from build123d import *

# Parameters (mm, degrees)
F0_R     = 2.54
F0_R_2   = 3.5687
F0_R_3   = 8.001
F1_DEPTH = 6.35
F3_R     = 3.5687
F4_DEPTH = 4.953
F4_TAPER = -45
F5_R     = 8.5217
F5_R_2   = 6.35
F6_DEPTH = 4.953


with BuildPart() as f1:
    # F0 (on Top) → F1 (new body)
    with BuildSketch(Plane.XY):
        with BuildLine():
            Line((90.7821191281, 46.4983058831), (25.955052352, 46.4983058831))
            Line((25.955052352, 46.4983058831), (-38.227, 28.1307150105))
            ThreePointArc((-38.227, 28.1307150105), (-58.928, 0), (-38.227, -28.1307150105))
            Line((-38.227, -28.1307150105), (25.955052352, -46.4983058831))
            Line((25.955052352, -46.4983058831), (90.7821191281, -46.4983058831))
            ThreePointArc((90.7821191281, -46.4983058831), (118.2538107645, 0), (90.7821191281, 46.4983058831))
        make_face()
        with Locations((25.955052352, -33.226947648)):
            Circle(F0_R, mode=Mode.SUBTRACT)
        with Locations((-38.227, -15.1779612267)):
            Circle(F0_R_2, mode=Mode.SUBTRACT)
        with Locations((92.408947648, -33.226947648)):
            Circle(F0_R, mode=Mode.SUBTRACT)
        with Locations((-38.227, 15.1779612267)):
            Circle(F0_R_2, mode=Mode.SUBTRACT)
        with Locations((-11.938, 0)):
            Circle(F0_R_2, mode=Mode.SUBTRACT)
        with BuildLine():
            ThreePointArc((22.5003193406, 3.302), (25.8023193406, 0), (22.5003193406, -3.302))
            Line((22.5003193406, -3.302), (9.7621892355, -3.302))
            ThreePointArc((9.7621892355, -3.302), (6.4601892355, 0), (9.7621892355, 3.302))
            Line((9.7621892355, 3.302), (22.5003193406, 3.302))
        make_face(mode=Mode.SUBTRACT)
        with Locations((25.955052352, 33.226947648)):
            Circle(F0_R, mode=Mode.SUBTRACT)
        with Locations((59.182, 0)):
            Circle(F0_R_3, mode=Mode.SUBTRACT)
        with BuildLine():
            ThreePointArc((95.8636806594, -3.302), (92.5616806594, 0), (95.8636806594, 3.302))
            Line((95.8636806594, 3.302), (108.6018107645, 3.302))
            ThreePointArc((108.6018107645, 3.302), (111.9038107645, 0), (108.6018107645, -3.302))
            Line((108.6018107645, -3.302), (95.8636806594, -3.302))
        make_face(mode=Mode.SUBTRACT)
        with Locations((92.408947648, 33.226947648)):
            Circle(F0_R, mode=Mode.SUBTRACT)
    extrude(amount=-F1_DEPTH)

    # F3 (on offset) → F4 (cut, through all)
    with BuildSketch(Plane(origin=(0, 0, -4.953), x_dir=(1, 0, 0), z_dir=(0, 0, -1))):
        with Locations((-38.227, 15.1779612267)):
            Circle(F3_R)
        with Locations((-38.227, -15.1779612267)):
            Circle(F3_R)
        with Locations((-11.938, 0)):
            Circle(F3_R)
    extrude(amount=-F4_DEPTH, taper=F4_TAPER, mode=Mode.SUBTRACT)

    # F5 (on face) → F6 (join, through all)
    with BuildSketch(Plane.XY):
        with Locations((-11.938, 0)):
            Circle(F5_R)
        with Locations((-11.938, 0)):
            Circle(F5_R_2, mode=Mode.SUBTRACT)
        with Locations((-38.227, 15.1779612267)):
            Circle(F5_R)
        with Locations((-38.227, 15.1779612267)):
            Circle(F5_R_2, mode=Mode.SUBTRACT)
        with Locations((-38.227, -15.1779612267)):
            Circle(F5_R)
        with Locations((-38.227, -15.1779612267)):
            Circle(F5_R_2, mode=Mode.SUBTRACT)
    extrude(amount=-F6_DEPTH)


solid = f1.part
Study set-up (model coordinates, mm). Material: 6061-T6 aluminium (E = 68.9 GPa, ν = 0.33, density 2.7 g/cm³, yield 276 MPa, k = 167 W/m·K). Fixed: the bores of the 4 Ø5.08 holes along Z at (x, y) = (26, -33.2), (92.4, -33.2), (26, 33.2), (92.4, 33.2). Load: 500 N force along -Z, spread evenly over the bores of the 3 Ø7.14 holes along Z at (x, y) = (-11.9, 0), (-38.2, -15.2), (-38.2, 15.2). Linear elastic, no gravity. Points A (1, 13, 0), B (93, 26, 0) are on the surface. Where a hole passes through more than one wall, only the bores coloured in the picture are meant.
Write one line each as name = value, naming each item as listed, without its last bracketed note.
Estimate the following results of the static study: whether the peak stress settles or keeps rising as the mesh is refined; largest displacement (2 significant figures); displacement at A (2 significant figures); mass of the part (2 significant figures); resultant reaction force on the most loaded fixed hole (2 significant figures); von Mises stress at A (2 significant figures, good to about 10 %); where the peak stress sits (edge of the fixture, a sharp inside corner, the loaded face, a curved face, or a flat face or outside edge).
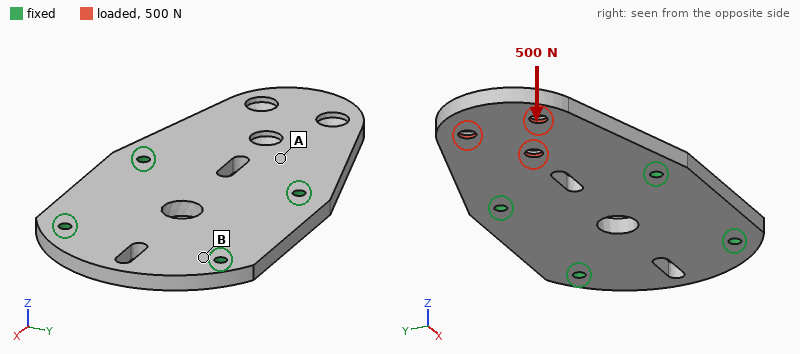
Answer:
whether the peak stress settles or keeps rising as the mesh is refined = keeps rising
largest displacement = 0.56 mm
displacement at A = 0.095 mm
mass of the part = 220 g
resultant reaction force on the most loaded fixed hole = 320 N
von Mises stress at A = 29 MPa
where the peak stress sits = edge of the fixture
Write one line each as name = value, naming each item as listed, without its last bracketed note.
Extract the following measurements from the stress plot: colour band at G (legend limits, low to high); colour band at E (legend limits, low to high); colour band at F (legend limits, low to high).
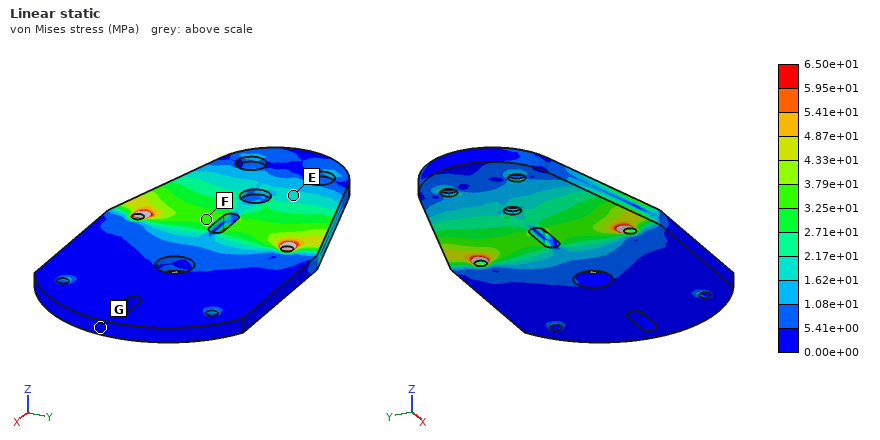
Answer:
colour band at G = 0.00e+00 to 5.41e+00 MPa
colour band at E = 1.62e+01 to 2.17e+01 MPa
colour band at F = 3.25e+01 to 3.79e+01 MPa
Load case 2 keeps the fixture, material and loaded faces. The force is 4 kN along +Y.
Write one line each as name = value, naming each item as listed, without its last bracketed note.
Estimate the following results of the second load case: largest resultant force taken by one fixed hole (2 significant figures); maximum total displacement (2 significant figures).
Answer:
largest resultant force taken by one fixed hole = 3.5 kN
maximum total displacement = 80 µm
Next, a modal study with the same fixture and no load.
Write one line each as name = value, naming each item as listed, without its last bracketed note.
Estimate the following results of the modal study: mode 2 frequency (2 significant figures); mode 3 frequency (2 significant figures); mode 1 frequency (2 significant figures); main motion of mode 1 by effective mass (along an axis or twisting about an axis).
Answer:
mode 2 frequency = 3000 Hz
mode 3 frequency = 4300 Hz
mode 1 frequency = 880 Hz
main motion of mode 1 by effective mass = along Z
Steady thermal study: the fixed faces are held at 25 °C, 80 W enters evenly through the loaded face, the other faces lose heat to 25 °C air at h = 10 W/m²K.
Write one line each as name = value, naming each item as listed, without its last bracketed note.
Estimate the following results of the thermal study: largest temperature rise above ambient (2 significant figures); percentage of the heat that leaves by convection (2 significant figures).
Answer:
largest temperature rise above ambient = 78 K
percentage of the heat that leaves by convection = 7.0 %
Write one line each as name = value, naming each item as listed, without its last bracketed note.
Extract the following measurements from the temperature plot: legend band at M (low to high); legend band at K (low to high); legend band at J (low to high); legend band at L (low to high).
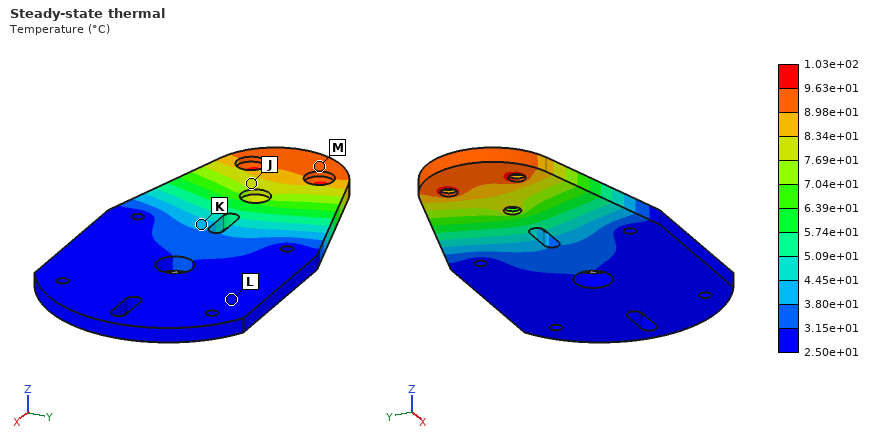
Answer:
legend band at M = 8.98e+01 to 9.63e+01 °C
legend band at K = 3.80e+01 to 4.45e+01 °C
legend band at J = 7.69e+01 to 8.34e+01 °C
legend band at L = 2.50e+01 to 3.15e+01 °C
